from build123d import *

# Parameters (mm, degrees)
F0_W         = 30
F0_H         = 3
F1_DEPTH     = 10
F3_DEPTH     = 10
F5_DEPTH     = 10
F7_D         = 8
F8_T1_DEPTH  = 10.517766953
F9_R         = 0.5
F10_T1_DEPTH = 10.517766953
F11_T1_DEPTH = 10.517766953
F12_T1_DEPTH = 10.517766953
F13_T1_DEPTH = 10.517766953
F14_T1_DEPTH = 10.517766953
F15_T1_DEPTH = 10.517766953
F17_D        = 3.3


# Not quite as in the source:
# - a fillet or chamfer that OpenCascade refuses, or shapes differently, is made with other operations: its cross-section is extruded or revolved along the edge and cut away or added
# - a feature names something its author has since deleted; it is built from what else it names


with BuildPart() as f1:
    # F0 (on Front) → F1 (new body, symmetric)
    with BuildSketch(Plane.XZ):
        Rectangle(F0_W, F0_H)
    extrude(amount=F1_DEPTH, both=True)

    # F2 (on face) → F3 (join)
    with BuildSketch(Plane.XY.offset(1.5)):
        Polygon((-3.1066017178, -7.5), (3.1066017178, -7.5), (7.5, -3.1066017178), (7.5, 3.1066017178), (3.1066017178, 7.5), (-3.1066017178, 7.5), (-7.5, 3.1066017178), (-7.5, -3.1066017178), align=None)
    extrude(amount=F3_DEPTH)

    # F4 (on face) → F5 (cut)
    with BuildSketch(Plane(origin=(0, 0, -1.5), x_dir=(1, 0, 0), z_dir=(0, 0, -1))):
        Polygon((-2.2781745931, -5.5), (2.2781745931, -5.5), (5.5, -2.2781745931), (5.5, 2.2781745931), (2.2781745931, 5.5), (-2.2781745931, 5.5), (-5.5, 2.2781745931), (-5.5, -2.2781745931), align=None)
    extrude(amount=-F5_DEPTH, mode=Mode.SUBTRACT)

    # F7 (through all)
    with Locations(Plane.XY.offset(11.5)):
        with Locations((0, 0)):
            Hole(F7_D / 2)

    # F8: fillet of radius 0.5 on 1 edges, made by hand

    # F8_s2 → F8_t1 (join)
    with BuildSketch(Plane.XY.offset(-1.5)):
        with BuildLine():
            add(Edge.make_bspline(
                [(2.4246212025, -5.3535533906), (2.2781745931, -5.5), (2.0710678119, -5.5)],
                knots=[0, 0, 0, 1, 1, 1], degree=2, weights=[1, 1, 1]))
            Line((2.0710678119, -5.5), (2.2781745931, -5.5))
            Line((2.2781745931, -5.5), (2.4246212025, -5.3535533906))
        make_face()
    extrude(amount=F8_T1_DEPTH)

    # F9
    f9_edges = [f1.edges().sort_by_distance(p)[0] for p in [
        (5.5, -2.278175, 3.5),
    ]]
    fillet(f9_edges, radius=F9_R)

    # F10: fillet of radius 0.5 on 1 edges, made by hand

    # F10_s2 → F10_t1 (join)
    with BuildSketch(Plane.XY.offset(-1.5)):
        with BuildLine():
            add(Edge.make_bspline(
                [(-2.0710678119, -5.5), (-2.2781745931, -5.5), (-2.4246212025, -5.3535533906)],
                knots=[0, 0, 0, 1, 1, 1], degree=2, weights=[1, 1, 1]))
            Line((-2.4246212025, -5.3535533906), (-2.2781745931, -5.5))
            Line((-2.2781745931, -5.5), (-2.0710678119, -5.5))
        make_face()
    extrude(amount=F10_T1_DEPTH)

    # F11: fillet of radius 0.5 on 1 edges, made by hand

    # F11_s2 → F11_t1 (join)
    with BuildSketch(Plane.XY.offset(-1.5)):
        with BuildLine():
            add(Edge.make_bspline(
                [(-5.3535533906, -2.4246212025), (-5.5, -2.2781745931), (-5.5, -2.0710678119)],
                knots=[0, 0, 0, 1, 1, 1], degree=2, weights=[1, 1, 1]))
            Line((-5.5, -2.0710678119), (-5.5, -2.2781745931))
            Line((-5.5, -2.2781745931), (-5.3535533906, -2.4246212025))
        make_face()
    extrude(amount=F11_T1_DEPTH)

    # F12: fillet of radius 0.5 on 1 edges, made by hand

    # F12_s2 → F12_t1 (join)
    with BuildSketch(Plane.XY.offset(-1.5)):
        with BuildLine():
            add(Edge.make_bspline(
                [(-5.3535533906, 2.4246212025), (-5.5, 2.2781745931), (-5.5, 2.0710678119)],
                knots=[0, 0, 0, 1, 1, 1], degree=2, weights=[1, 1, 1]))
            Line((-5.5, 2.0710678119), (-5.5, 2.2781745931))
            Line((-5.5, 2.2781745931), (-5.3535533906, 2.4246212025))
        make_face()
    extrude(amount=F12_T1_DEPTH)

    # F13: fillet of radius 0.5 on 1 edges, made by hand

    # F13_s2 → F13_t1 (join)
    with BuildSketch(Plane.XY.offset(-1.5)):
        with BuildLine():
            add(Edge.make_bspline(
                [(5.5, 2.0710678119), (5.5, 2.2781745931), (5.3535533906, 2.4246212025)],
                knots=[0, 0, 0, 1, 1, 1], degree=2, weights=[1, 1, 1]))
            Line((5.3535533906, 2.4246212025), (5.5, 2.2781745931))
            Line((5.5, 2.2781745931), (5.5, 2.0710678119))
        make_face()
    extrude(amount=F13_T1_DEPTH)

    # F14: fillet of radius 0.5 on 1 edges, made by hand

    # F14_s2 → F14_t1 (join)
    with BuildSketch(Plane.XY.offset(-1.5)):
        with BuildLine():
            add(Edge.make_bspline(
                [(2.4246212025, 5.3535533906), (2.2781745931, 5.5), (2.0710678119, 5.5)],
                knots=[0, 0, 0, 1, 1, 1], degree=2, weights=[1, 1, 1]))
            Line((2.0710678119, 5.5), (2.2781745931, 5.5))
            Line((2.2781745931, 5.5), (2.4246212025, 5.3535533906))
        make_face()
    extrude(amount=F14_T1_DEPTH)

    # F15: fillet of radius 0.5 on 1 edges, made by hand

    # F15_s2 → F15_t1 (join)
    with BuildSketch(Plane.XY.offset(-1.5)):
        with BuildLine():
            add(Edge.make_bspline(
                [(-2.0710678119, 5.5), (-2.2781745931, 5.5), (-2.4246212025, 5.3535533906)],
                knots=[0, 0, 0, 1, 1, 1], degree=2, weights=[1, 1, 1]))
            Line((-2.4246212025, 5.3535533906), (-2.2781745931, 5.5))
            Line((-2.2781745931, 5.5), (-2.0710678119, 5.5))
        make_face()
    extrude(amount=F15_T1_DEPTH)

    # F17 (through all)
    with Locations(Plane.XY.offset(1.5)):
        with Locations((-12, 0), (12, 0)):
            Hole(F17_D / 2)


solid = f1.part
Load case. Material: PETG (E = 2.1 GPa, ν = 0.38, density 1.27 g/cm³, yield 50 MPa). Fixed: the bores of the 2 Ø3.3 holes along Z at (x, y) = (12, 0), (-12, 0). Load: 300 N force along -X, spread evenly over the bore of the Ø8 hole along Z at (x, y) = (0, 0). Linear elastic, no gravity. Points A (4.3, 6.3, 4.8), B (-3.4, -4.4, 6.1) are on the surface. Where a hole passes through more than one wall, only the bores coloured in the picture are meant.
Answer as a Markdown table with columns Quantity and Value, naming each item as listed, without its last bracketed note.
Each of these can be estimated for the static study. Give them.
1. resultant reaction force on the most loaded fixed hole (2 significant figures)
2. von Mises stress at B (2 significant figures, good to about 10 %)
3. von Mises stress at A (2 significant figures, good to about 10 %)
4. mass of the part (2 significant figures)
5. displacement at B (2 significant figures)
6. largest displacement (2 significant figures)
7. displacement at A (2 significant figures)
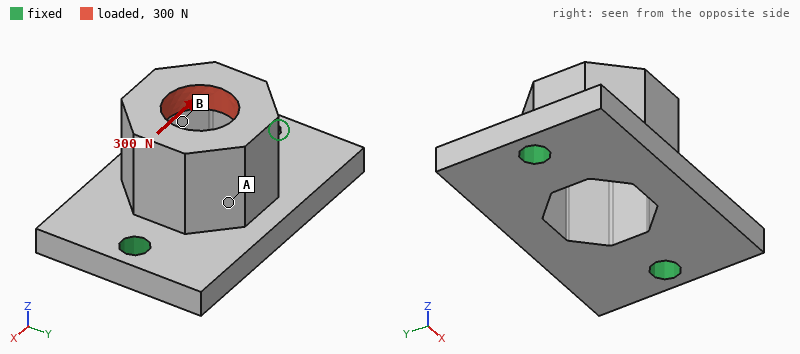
| Quantity | Value |
|---|---|
| resultant reaction force on the most loaded fixed hole | 220 N |
| von Mises stress at B | 12 MPa |
| von Mises stress at A | 6.6 MPa |
| mass of the part | 3.1 g |
| displacement at B | 0.11 mm |
| largest displacement | 0.24 mm |
| displacement at A | 0.097 mm |
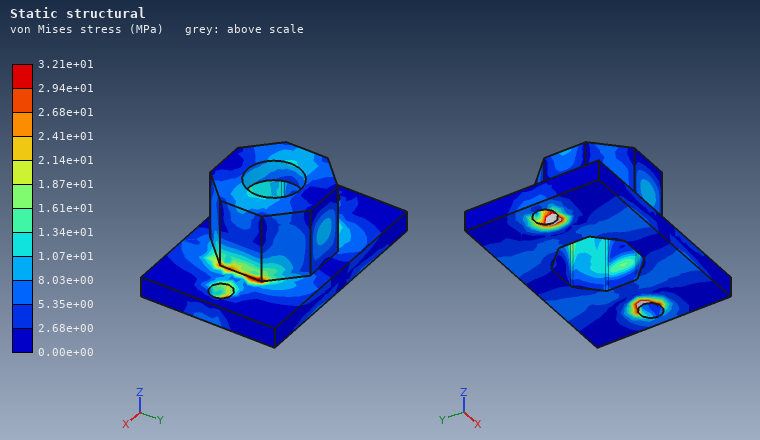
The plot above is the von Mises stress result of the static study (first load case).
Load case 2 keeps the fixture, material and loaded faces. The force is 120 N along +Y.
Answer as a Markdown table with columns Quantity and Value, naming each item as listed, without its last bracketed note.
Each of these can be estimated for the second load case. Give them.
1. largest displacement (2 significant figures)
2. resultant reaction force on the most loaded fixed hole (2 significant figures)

| Quantity | Value |
|---|---|
| largest displacement | 0.46 mm |
| resultant reaction force on the most loaded fixed hole | 60 N |
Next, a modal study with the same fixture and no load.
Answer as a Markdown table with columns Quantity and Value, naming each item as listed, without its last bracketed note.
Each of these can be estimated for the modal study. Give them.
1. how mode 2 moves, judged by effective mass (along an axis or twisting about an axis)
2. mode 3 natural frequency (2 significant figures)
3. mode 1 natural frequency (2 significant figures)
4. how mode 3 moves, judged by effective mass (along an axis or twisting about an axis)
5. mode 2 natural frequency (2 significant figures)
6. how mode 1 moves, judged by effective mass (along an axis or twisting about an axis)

| Quantity | Value |
|---|---|
| how mode 2 moves, judged by effective mass | along Z |
| mode 3 natural frequency | 6600 Hz |
| mode 1 natural frequency | 2600 Hz |
| how mode 3 moves, judged by effective mass | along X |
| mode 2 natural frequency | 5700 Hz |
| how mode 1 moves, judged by effective mass | along Y |
